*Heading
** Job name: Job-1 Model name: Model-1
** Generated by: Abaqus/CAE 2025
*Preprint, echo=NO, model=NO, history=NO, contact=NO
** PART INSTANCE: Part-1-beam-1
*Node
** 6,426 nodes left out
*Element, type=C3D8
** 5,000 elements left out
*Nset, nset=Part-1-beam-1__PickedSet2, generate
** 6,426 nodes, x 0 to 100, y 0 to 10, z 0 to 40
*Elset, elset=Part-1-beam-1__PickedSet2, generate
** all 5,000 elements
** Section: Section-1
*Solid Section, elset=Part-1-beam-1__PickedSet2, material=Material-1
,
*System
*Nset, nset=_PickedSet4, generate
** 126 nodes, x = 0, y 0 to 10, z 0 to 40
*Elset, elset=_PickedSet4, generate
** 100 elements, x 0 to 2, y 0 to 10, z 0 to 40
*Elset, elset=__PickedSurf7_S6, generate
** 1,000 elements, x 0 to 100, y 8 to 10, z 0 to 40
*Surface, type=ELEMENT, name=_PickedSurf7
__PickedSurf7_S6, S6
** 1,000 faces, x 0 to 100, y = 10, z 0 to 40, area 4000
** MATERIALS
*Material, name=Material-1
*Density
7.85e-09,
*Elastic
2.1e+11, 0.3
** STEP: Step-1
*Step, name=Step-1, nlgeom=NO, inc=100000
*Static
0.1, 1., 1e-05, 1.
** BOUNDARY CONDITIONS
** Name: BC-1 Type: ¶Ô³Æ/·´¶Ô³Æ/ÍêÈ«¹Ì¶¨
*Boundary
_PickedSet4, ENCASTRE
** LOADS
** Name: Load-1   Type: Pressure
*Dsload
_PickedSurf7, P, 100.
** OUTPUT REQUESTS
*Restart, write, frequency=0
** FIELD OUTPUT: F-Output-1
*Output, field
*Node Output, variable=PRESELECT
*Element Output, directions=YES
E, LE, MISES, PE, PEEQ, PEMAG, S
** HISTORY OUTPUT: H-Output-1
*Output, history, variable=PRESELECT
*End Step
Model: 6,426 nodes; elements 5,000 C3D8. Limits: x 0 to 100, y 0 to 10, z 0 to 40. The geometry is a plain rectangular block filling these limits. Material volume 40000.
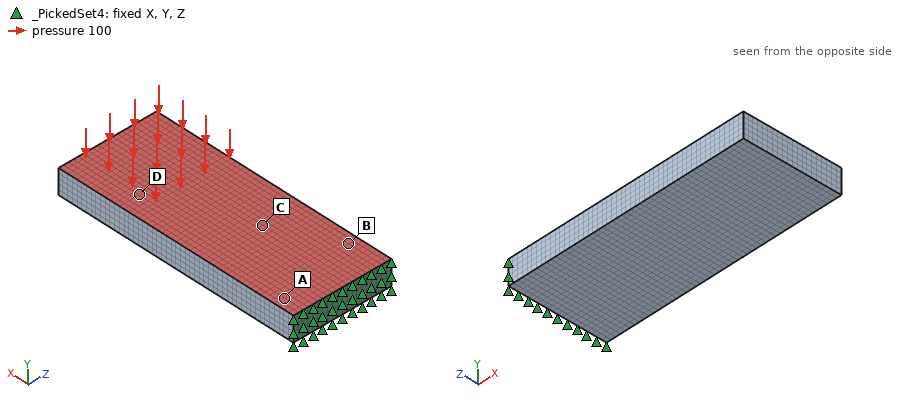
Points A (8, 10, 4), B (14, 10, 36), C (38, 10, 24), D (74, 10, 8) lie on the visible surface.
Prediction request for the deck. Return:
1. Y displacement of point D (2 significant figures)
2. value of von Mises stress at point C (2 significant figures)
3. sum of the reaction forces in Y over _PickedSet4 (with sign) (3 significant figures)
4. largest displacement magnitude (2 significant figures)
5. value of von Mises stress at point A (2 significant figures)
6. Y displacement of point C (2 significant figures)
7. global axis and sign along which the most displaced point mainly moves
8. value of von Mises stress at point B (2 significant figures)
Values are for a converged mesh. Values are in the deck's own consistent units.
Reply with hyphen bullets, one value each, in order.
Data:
- -4.6e-05
- 11000
- 4.00e+05
- 7.0e-05
- 25000
- -1.6e-05
- -Y
- 22000
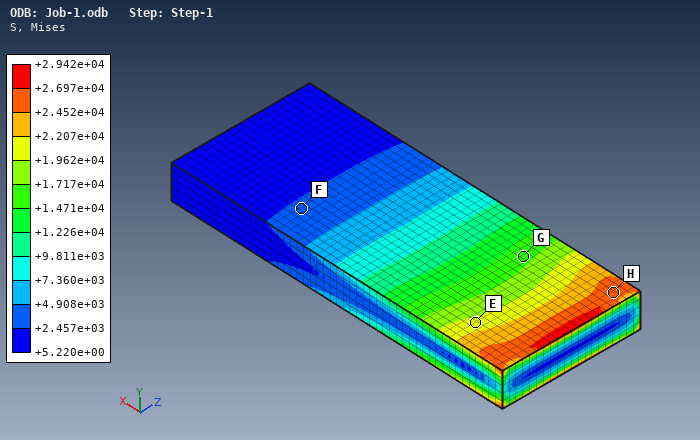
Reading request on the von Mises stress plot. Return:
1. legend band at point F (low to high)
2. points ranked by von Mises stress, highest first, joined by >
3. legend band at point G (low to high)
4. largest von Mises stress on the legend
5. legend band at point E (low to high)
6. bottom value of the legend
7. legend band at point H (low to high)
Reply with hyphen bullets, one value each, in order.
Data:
- +2.457e+03 to +4.908e+03
- H > E > G > F
- +1.471e+04 to +1.717e+04
- +2.942e+04
- +1.962e+04 to +2.207e+04
- +5.220e+00
- +2.452e+04 to +2.697e+04
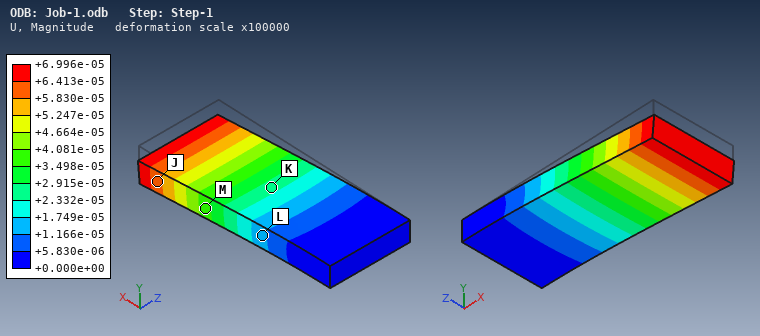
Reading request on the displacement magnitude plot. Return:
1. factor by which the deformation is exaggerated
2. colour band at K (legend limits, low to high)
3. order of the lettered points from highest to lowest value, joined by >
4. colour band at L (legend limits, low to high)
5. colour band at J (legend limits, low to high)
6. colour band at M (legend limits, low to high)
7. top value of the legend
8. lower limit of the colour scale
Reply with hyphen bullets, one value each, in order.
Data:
- 100000
- +2.332e-05 to +2.915e-05
- J > M > K > L
- +1.166e-05 to +1.749e-05
- +5.830e-05 to +6.413e-05
- +3.498e-05 to +4.081e-05
- +6.996e-05
- +0.000e+00
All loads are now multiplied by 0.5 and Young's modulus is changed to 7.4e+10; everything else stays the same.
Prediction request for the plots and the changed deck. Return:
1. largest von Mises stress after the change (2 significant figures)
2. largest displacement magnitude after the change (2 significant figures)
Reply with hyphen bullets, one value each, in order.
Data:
- 15000
- 9.9e-05
